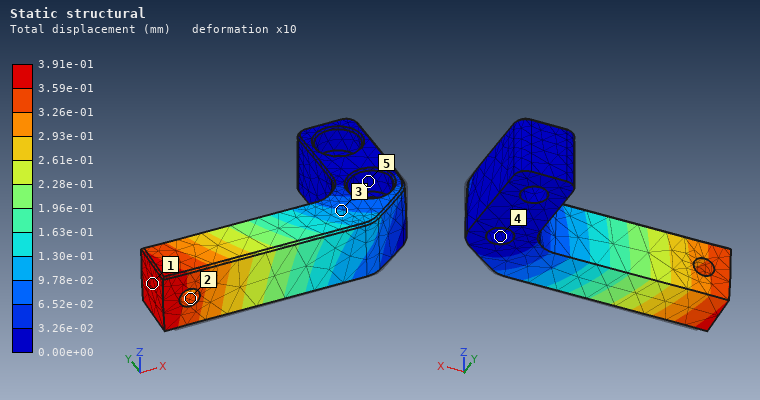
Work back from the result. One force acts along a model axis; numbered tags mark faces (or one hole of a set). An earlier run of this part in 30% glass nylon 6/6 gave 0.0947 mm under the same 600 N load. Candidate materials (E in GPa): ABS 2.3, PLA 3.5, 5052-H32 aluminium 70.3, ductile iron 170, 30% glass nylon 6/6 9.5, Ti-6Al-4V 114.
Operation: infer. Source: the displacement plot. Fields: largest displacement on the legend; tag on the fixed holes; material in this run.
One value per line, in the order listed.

3.91e-01 mm
4
ABS
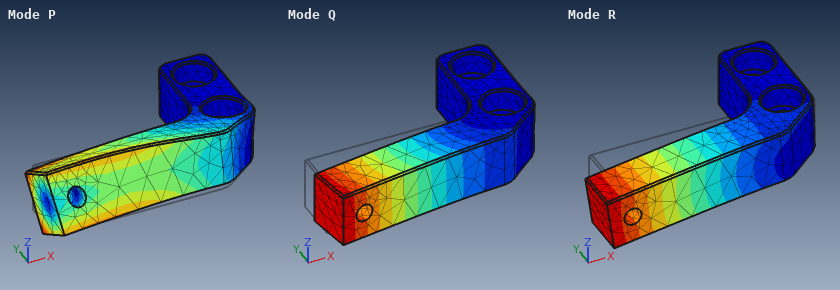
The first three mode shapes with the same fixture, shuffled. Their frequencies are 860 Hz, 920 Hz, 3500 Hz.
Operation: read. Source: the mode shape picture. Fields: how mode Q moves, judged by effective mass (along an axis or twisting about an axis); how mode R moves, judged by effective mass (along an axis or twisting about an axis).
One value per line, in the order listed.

along Y
along Z
